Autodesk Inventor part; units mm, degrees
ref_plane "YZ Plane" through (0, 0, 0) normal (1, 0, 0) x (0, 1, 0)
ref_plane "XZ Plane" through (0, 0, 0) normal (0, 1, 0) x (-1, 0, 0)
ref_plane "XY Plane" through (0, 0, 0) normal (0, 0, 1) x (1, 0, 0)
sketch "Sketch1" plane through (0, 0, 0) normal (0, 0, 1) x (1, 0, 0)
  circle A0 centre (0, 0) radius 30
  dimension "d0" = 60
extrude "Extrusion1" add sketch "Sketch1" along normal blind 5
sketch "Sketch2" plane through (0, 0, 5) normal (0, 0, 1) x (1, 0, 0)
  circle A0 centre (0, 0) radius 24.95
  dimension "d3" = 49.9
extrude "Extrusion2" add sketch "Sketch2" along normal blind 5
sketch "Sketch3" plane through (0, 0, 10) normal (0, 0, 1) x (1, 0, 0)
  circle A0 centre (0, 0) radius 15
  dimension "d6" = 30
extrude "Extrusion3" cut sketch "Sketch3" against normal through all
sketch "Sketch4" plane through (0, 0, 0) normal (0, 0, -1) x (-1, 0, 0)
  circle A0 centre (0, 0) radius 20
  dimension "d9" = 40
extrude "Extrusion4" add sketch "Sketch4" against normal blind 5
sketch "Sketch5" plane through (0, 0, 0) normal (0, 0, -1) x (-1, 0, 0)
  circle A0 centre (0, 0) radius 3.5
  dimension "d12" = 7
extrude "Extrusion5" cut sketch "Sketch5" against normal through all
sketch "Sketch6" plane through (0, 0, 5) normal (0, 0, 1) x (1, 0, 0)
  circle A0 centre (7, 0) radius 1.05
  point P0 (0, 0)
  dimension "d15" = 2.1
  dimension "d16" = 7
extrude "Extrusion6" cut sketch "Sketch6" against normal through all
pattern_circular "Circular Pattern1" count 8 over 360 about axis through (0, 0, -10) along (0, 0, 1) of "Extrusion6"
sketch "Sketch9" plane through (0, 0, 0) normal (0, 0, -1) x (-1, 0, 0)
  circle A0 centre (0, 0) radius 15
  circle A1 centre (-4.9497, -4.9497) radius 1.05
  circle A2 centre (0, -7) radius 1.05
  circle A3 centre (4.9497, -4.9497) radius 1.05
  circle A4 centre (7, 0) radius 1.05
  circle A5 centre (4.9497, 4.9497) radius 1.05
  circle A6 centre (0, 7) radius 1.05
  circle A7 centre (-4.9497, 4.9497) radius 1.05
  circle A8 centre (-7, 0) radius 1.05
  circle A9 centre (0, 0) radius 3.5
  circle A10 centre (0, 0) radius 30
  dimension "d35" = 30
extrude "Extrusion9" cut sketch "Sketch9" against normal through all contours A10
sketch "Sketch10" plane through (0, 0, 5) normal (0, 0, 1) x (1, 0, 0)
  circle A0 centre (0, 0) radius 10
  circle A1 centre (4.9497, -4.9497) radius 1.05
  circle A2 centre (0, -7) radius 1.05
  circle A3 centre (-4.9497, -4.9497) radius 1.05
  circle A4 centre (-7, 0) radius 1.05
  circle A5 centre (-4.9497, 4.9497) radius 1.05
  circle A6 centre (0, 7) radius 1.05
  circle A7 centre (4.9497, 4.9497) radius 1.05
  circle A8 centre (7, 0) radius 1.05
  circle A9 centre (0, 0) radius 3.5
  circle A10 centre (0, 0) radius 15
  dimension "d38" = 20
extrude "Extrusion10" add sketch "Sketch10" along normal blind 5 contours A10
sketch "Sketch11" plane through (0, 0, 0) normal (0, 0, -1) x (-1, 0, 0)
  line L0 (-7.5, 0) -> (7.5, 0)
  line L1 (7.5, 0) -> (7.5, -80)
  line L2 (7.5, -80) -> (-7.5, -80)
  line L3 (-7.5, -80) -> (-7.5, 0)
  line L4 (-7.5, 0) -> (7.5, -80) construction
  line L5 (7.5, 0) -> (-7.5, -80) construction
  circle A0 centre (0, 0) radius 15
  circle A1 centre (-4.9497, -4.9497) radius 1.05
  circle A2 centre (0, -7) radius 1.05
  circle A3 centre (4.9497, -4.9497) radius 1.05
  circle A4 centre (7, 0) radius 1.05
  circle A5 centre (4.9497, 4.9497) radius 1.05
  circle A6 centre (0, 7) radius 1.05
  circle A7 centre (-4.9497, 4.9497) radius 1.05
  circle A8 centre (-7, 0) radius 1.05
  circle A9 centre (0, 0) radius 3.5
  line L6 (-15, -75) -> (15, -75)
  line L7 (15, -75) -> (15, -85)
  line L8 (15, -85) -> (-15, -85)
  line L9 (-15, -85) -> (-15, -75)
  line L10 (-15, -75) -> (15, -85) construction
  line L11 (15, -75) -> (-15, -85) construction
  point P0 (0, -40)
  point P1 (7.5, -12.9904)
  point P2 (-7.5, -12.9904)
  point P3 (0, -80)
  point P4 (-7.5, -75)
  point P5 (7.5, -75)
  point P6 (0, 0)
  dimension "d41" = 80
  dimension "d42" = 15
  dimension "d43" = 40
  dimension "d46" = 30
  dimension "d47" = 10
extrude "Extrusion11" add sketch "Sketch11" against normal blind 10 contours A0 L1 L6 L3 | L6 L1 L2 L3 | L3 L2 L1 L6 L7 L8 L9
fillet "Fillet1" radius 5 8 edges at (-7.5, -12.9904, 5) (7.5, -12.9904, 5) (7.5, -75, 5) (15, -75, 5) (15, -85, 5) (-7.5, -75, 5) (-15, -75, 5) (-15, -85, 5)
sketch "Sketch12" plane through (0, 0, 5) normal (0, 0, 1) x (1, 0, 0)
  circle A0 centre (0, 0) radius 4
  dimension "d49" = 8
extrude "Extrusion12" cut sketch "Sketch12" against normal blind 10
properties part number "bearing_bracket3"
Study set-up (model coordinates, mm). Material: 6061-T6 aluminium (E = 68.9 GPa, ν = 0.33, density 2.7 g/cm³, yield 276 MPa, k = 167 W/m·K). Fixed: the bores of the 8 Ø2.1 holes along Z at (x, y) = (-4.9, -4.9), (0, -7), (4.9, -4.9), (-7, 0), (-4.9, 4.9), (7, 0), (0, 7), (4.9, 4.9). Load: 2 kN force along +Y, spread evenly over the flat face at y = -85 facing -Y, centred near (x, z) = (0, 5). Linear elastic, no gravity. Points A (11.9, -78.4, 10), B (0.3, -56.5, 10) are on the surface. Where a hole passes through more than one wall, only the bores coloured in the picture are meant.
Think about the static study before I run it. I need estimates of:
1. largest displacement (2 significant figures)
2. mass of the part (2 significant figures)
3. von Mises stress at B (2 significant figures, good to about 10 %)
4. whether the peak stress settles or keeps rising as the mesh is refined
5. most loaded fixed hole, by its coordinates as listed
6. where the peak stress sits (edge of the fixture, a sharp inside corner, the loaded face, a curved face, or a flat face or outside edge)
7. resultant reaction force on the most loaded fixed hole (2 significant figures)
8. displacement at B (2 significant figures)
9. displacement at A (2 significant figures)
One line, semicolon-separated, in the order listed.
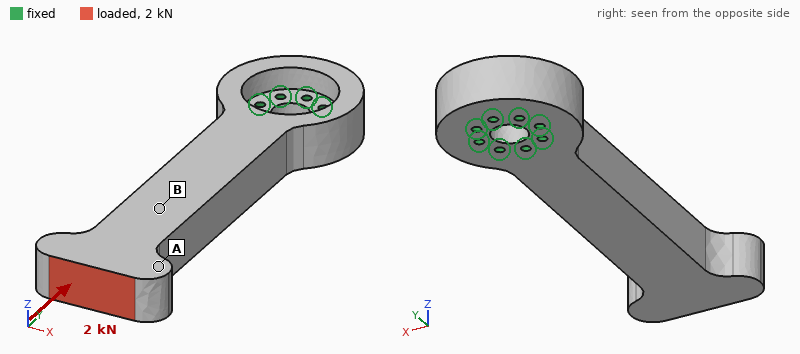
61 µm; 46 g; 13 MPa; keeps rising; (0, -7); edge of the fixture; 590 N; 40 µm; 56 µm
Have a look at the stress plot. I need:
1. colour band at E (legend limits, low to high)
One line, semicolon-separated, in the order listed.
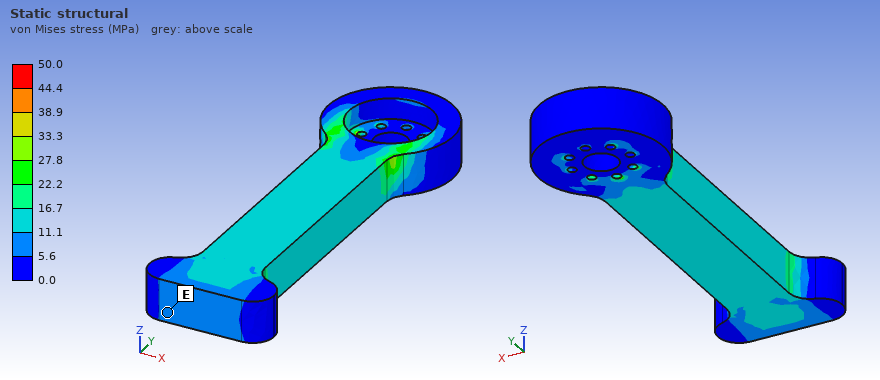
5.6 to 11.1 MPa
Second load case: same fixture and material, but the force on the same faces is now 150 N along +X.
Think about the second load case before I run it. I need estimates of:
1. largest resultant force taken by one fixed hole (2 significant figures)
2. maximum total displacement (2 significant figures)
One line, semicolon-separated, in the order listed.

490 N; 0.13 mm
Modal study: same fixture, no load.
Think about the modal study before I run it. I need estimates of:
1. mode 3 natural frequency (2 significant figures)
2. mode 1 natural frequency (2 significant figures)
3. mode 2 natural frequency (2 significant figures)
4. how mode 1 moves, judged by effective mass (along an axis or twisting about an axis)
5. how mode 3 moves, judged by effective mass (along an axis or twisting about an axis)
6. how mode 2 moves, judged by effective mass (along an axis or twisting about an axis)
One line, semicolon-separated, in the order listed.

5600 Hz; 930 Hz; 1600 Hz; along Z; twisting about Y; along X
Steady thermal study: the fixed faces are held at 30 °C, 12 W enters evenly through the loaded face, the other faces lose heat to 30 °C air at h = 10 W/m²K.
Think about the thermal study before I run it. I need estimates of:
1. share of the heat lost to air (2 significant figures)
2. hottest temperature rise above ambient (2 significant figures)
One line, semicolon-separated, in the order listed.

7.2 %; 35 K
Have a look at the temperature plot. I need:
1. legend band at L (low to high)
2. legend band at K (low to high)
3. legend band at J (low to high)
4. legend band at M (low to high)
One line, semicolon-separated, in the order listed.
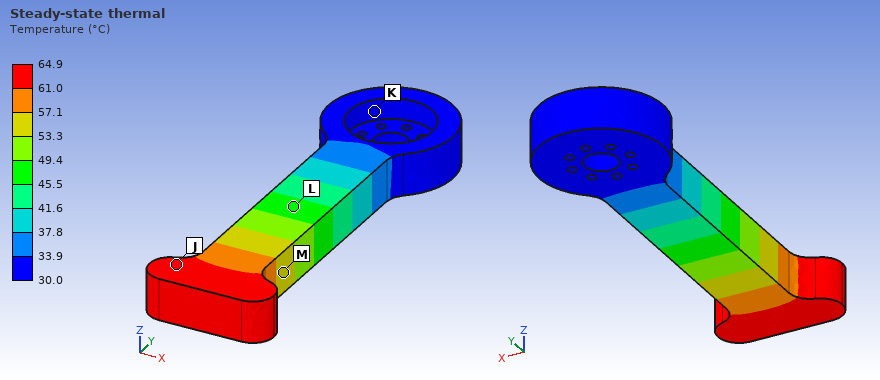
45.5 to 49.4 °C; 30.0 to 33.9 °C; 61.0 to 64.9 °C; 53.3 to 57.1 °C
